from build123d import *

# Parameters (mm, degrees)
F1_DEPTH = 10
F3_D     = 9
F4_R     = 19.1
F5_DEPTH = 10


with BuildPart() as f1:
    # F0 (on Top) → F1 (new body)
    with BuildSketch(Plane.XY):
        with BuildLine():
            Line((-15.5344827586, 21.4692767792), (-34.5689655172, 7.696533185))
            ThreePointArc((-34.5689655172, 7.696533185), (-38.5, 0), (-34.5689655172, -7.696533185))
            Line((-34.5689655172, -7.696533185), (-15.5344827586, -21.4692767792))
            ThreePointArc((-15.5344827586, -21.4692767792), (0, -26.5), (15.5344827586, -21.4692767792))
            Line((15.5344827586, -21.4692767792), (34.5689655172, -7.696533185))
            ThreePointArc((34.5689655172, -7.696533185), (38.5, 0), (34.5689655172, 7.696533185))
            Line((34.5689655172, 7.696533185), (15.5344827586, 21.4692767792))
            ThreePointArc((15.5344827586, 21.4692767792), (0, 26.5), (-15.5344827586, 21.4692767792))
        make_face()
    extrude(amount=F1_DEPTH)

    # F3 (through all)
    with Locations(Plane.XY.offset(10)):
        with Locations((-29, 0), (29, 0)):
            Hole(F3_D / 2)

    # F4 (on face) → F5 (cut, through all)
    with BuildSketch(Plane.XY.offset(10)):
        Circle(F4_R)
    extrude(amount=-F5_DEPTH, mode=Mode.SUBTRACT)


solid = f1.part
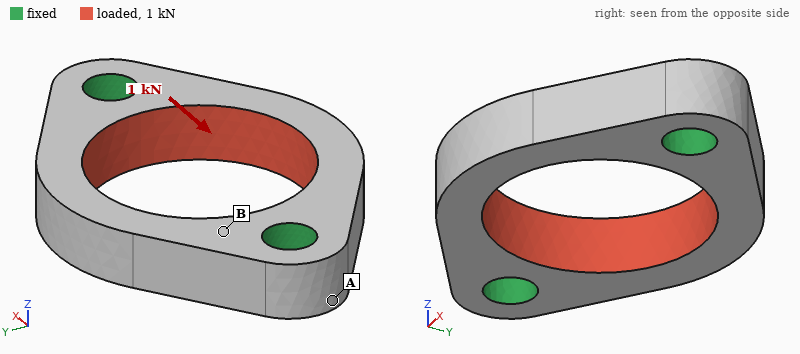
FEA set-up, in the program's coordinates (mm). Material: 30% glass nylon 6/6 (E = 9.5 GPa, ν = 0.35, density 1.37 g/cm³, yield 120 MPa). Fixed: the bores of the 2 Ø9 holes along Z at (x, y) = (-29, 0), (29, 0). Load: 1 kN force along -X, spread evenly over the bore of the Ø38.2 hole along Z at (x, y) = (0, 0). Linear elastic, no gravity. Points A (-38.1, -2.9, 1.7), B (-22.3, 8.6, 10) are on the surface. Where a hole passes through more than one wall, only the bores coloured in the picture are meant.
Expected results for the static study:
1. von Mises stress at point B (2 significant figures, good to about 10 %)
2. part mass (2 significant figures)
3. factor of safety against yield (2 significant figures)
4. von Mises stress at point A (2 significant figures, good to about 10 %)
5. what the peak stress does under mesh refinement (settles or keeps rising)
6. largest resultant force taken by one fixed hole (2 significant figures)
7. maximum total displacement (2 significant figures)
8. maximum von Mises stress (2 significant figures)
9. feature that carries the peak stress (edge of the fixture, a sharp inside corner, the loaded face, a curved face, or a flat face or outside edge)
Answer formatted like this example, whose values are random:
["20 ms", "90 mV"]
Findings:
["2.9 MPa", "20 g", "21", "1.4 MPa", "settles", "500 N", "16 µm", "5.6 MPa", "the loaded face"]
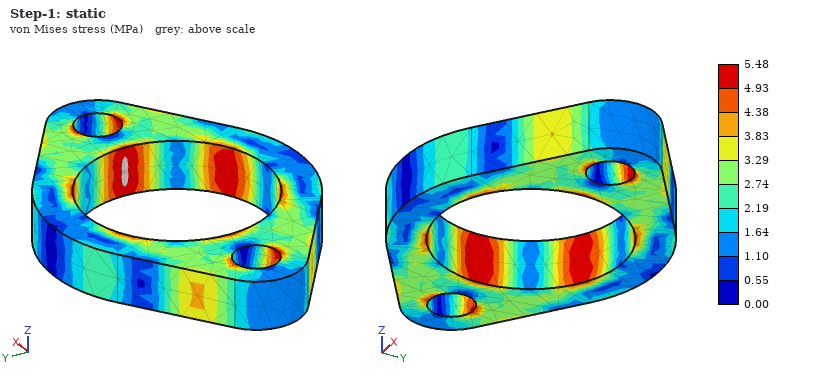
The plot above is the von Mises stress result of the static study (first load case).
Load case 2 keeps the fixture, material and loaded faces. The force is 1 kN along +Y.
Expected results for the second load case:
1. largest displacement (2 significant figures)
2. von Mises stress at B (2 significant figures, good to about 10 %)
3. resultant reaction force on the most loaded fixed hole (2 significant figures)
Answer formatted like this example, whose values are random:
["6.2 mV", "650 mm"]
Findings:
["14 µm", "2.9 MPa", "500 N"]
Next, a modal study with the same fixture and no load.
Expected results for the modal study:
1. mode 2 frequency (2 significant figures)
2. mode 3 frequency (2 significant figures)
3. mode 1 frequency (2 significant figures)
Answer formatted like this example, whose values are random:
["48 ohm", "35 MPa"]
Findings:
["4900 Hz", "9700 Hz", "4700 Hz"]
